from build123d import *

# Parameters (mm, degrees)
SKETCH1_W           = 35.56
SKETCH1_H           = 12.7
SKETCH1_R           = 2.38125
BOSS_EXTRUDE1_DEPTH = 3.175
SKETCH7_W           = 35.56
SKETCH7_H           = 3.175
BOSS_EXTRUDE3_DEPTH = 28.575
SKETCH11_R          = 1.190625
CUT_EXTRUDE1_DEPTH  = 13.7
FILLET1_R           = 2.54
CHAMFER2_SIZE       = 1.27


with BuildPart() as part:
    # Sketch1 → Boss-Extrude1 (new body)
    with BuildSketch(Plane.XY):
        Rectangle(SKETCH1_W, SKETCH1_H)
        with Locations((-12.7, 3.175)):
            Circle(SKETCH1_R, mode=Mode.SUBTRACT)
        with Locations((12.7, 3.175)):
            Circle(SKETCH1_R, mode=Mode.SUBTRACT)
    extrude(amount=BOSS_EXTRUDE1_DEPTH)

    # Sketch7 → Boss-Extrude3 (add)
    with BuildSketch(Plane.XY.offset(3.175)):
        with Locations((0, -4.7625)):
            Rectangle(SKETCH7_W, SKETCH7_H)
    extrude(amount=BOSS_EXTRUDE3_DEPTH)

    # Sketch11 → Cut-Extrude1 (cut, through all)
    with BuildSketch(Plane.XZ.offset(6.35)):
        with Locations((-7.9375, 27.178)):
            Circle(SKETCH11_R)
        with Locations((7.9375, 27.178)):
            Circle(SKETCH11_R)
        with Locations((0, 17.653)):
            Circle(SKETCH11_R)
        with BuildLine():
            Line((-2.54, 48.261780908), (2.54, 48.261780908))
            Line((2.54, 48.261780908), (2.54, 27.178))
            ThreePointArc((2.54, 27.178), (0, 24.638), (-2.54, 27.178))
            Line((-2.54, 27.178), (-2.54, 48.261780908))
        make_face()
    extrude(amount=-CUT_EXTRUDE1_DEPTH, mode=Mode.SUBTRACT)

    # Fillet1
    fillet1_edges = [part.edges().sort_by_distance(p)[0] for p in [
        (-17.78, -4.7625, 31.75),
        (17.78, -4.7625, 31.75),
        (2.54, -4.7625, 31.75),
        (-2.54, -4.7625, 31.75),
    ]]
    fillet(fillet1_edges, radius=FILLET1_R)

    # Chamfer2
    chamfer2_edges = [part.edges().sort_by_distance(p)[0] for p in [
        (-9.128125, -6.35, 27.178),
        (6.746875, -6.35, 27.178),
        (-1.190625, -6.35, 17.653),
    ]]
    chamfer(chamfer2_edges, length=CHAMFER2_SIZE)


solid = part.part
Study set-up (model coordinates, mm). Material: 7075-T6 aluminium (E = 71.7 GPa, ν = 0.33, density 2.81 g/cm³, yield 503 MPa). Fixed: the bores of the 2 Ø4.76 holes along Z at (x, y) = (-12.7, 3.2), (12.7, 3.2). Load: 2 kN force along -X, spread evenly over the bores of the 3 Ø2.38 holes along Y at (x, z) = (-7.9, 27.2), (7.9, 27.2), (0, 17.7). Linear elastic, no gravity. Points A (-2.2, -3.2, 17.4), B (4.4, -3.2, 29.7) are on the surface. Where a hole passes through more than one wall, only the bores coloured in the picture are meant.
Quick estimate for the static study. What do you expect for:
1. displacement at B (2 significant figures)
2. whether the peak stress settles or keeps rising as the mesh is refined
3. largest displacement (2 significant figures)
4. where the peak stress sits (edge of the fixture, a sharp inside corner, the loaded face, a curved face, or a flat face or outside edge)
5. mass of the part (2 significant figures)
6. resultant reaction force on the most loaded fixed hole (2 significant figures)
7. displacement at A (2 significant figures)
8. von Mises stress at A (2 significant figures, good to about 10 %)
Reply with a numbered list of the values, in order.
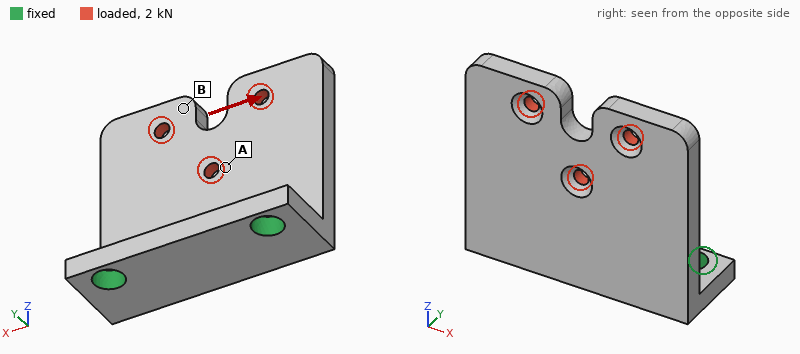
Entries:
1. 0.17 mm
2. keeps rising
3. 0.23 mm
4. edge of the fixture
5. 12 g
6. 2.0 kN
7. 0.096 mm
8. 110 MPa
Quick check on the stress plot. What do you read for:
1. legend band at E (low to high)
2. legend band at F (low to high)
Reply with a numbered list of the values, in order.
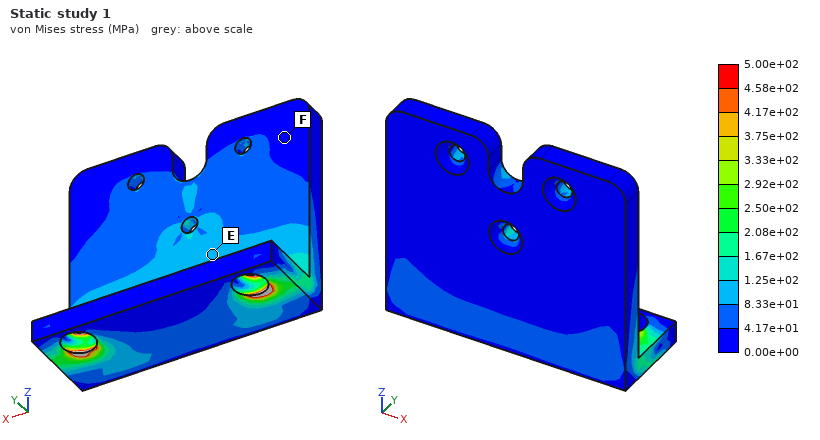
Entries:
1. 8.33e+01 to 1.25e+02 MPa
2. 0.00e+00 to 4.17e+01 MPa
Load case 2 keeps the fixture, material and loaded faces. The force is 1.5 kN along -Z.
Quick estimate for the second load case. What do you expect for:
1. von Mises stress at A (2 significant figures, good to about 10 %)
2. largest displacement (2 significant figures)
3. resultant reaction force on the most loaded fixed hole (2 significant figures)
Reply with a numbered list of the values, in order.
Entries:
1. 32 MPa
2. 0.11 mm
3. 750 N
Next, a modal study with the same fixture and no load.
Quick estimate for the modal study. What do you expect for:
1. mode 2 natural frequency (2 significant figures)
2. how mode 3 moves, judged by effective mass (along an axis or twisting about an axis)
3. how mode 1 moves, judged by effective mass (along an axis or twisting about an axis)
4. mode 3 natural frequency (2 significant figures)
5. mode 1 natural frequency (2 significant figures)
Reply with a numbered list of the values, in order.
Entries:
1. 5000 Hz
2. along X
3. along Y
4. 8700 Hz
5. 2300 Hz
